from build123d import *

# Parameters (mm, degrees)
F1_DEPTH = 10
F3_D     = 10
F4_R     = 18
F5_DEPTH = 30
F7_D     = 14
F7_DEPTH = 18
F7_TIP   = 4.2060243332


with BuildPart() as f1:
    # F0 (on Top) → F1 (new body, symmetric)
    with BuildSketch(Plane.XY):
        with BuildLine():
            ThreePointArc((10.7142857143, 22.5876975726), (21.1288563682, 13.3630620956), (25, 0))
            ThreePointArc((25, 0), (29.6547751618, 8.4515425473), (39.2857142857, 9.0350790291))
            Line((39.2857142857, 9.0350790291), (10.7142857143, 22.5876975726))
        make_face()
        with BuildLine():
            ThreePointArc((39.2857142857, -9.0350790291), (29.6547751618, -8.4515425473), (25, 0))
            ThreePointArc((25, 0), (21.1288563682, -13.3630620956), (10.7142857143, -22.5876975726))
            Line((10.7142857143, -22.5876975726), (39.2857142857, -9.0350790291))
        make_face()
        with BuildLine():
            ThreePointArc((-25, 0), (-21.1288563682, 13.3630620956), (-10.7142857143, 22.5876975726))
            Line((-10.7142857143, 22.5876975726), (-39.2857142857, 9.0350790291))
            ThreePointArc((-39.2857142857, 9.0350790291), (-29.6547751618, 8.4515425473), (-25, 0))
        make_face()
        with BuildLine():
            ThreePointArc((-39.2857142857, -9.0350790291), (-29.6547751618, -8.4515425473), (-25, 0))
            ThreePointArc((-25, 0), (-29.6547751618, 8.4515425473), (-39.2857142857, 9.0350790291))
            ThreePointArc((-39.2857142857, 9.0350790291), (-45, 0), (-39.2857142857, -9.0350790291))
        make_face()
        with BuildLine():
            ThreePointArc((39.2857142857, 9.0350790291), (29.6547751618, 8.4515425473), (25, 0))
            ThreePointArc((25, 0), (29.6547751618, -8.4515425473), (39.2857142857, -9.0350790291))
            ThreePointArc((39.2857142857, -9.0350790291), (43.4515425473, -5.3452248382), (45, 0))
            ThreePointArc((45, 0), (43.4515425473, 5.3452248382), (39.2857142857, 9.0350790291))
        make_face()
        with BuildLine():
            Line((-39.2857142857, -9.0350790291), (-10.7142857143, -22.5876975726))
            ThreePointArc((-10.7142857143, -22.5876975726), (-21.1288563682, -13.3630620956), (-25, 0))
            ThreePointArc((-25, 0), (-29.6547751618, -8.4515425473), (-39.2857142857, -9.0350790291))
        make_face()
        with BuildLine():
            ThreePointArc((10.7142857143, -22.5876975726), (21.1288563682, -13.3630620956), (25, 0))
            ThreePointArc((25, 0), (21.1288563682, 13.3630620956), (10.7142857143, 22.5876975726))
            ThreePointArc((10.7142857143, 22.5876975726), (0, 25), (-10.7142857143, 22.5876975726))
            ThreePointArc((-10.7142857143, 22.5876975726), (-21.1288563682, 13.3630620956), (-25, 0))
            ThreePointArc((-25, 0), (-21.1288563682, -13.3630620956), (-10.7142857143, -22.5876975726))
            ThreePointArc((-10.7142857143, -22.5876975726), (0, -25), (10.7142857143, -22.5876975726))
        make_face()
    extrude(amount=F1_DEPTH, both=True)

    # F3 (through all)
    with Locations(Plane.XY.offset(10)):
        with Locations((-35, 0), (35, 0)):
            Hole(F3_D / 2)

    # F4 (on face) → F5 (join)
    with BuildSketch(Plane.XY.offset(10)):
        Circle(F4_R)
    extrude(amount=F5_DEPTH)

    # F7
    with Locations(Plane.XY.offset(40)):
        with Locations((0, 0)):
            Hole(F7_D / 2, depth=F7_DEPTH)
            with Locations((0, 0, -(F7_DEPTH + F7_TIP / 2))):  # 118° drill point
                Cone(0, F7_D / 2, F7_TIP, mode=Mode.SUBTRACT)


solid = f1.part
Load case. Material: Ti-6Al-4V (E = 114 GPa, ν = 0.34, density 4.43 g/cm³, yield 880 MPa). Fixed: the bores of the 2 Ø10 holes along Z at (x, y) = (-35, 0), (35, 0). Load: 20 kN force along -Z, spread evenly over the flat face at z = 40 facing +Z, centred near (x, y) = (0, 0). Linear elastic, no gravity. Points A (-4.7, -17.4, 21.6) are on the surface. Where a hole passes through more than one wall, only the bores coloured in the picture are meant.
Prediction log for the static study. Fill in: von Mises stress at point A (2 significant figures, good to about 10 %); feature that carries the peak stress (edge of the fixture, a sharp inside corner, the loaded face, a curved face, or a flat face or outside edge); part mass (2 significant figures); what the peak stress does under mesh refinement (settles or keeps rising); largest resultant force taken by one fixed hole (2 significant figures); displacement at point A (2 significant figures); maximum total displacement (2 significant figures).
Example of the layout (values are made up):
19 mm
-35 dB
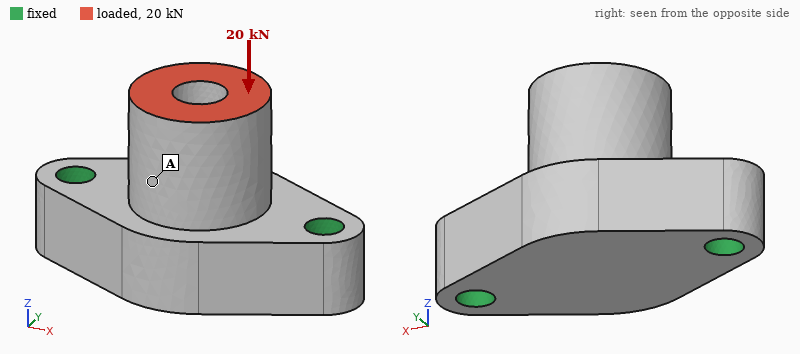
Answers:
17 MPa
edge of the fixture
370 g
keeps rising
10 kN
17 µm
21 µm
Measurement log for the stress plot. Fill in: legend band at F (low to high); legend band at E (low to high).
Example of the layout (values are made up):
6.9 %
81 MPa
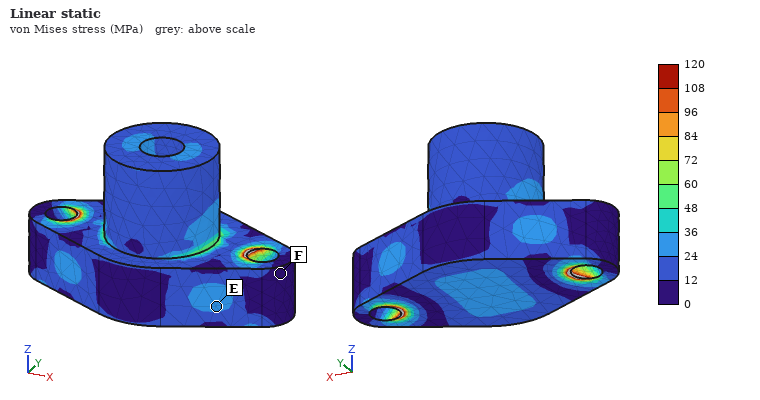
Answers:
0 to 12 MPa
24 to 36 MPa
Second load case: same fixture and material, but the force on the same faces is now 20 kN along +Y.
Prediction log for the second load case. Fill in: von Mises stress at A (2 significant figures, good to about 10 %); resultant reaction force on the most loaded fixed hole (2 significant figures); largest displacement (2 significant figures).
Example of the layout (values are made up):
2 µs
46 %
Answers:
88 MPa
10 kN
0.23 mm
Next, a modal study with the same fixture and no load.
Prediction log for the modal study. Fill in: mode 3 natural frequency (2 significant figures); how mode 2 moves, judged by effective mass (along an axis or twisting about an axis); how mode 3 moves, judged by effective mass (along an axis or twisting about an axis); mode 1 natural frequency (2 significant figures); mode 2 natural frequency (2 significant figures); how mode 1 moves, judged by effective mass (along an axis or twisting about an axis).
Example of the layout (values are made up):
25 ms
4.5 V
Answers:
12 kHz
along Z
along X
6000 Hz
11 kHz
along Y
